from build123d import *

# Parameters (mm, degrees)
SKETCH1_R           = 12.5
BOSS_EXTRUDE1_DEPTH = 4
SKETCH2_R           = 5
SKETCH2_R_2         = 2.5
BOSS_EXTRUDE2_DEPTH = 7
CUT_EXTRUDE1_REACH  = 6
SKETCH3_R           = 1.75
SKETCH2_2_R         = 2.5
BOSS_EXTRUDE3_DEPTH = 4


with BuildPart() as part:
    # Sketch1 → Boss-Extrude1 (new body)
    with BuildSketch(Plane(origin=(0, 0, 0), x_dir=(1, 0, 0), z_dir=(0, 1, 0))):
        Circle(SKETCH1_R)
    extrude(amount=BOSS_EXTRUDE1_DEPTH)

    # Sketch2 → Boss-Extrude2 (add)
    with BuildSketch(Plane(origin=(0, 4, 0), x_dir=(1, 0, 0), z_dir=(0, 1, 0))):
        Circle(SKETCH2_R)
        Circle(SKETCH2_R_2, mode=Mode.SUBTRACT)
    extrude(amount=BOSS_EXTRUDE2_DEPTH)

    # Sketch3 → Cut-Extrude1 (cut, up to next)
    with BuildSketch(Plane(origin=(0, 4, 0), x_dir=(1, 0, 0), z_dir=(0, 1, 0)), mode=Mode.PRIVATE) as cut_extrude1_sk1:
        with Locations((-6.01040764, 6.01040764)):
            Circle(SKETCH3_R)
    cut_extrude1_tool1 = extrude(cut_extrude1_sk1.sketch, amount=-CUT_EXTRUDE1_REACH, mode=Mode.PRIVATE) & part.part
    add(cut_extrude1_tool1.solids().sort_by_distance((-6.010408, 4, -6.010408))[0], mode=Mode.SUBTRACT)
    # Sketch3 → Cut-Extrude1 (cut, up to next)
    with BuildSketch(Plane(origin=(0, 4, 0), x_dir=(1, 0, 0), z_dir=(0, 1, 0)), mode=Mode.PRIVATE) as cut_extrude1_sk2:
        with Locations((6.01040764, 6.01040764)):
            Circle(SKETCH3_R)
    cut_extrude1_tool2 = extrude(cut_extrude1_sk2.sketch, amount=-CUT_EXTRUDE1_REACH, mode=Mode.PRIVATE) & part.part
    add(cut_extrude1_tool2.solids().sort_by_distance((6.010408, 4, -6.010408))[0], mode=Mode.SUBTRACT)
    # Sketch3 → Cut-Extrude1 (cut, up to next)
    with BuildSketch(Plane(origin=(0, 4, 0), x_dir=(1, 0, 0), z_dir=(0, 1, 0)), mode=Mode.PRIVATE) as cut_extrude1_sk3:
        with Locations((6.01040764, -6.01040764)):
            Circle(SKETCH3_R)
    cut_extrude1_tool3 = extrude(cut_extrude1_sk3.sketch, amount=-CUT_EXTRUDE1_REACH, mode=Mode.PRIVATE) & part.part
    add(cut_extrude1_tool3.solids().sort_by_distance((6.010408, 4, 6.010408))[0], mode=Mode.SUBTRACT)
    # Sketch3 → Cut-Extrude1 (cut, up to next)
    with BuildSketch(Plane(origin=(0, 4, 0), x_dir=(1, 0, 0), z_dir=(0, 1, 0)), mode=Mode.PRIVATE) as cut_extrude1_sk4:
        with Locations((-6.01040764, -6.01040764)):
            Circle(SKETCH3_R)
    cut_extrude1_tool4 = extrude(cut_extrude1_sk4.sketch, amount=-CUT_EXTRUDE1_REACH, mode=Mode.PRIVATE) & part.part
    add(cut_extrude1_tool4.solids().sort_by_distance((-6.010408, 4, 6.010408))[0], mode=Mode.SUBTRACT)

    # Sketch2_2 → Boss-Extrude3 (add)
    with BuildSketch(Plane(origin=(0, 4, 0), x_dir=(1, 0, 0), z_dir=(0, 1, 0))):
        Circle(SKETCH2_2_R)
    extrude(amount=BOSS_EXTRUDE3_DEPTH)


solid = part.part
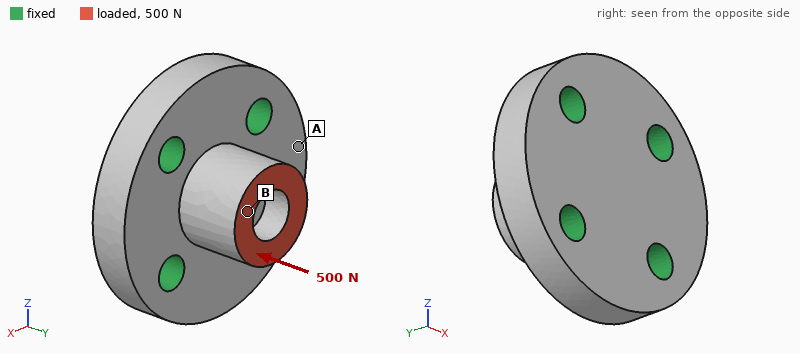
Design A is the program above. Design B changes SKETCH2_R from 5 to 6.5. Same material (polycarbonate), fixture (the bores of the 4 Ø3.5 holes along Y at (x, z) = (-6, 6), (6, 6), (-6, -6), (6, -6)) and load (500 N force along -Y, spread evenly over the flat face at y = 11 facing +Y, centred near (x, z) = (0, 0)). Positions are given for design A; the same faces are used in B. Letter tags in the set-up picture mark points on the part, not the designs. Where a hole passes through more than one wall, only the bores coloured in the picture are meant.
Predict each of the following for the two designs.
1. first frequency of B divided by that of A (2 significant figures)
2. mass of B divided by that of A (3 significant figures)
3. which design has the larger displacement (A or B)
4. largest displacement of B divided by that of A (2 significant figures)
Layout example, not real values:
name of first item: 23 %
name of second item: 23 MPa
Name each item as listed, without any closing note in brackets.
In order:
first frequency of B divided by that of A: 1.1
mass of B divided by that of A: 1.16
which design has the larger displacement: A
largest displacement of B divided by that of A: 0.53
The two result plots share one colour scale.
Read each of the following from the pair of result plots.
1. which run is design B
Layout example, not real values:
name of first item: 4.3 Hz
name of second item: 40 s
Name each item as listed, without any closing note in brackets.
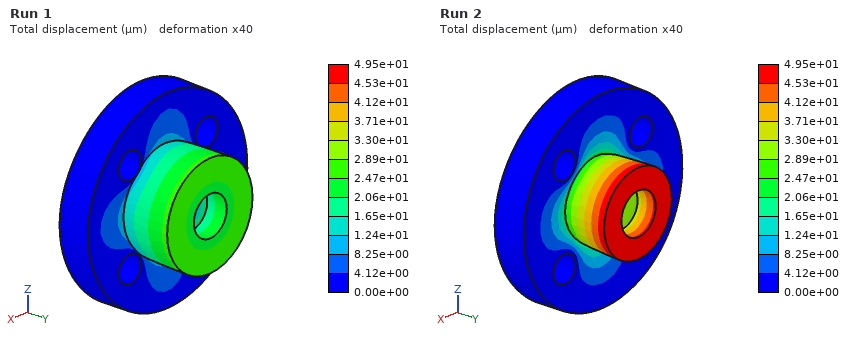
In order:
which run is design B: Run 1
